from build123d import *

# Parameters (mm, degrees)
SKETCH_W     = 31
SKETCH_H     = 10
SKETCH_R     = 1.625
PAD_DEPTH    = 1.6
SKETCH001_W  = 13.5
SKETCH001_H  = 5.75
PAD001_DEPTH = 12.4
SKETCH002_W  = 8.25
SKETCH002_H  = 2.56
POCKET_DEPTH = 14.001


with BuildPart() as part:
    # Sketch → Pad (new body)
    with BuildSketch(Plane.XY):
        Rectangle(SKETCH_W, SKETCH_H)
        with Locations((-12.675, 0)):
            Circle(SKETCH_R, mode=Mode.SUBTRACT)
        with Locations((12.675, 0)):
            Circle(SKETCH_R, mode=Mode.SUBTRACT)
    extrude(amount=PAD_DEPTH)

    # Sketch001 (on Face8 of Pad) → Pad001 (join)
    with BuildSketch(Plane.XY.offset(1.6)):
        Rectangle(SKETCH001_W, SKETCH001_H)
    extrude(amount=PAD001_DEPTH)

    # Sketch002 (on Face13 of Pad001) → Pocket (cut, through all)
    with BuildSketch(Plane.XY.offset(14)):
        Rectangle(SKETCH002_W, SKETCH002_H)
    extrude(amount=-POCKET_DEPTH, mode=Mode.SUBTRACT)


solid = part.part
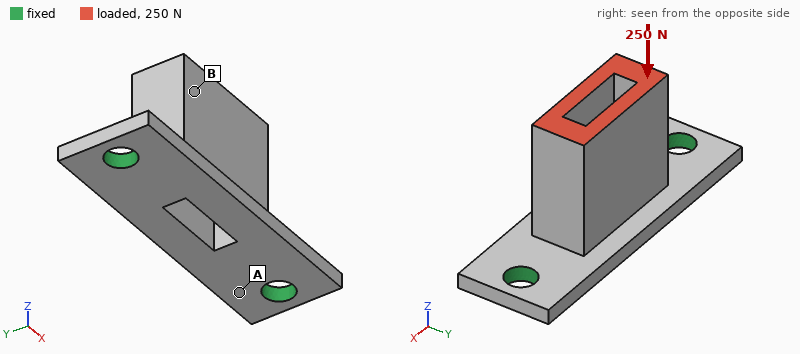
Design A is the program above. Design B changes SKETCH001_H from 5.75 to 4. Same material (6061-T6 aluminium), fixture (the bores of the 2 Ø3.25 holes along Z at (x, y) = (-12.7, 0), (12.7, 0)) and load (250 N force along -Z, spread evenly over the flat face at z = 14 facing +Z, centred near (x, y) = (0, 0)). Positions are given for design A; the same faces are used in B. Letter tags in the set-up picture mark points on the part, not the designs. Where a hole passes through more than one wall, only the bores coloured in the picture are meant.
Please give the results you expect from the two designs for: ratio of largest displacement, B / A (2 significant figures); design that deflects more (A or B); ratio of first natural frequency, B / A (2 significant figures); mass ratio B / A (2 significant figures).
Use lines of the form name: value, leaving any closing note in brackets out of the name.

ratio of largest displacement, B / A: 1.2
design that deflects more: B
ratio of first natural frequency, B / A: 1.2
mass ratio B / A: 0.74
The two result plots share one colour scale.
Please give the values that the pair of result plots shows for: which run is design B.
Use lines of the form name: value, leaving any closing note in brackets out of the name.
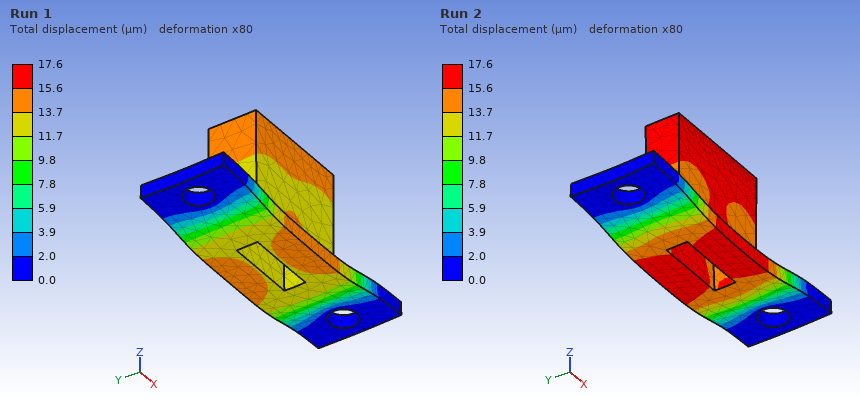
which run is design B: Run 2
